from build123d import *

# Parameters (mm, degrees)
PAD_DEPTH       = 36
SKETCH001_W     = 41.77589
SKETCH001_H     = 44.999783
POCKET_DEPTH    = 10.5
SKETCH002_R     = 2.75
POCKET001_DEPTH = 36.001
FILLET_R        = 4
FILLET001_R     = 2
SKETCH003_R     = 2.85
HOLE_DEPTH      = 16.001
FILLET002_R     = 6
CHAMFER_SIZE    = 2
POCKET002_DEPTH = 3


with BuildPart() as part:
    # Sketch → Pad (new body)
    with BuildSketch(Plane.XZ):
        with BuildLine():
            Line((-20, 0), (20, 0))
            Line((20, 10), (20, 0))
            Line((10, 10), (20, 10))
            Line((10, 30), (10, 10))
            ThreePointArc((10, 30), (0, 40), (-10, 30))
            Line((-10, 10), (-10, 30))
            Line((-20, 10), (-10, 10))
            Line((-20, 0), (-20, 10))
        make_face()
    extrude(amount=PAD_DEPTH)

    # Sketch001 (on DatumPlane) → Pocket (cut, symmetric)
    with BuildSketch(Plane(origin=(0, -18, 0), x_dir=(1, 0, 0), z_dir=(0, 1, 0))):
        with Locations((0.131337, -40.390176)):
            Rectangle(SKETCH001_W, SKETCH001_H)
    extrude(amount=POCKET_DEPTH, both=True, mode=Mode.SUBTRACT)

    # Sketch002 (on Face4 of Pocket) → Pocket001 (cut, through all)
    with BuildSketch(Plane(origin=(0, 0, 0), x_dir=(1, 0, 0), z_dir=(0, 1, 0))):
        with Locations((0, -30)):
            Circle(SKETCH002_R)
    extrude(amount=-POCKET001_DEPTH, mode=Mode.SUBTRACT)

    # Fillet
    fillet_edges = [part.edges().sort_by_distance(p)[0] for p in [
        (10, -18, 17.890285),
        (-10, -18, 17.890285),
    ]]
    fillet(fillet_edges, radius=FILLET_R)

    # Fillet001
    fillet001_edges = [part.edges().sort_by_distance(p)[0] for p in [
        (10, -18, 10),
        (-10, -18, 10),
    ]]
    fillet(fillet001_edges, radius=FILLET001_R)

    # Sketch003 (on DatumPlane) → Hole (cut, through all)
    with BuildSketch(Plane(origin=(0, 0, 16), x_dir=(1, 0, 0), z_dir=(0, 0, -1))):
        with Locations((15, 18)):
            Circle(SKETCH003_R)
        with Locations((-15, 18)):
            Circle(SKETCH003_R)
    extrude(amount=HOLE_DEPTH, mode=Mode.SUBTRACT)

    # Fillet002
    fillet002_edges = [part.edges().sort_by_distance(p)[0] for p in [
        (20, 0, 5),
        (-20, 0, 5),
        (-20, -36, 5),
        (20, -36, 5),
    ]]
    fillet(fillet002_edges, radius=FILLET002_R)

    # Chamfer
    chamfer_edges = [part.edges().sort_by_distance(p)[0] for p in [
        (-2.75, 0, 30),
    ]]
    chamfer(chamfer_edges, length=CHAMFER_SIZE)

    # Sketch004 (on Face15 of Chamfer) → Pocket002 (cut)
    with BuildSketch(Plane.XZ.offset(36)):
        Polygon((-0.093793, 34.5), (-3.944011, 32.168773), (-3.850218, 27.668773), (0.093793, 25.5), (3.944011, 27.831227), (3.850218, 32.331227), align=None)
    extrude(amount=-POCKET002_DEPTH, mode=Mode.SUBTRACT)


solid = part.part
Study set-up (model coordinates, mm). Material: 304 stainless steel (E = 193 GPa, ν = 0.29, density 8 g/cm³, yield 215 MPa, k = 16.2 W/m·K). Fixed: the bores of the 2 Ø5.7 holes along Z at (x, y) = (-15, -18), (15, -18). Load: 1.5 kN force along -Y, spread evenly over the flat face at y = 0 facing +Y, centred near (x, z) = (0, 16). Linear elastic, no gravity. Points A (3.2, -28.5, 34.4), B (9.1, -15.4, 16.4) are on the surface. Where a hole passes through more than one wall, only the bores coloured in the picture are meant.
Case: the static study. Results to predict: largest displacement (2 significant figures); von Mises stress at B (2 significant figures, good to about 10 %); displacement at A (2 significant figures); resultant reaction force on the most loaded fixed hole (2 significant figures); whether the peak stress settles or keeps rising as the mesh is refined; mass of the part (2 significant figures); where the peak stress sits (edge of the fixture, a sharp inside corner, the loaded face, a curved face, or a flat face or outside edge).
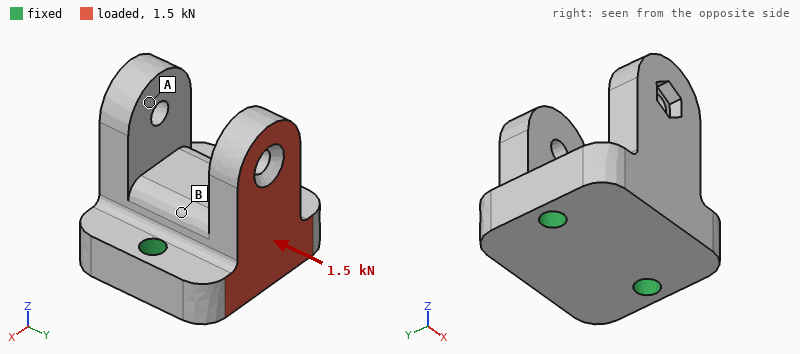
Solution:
19 µm
8.6 MPa
3.8 µm
750 N
keeps rising
200 g
edge of the fixture
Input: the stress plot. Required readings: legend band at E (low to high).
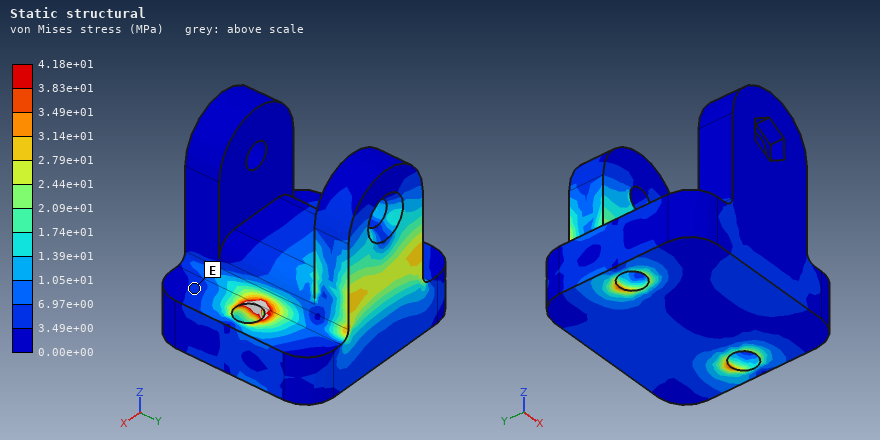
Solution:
3.49e+00 to 6.97e+00 MPa
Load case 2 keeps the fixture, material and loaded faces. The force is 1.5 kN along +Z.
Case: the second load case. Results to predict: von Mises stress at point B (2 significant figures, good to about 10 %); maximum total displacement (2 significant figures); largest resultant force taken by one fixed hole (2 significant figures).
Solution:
9.3 MPa
16 µm
800 N
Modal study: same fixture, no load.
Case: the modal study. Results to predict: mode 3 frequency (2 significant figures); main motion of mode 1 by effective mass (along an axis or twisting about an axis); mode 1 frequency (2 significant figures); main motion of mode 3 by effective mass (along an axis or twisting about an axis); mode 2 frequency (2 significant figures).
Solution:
12 kHz
along Y
6700 Hz
along X
9100 Hz
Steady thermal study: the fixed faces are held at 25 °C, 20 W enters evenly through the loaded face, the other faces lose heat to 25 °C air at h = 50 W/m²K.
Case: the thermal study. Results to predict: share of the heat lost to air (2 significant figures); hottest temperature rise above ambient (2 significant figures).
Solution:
29 %
74 K
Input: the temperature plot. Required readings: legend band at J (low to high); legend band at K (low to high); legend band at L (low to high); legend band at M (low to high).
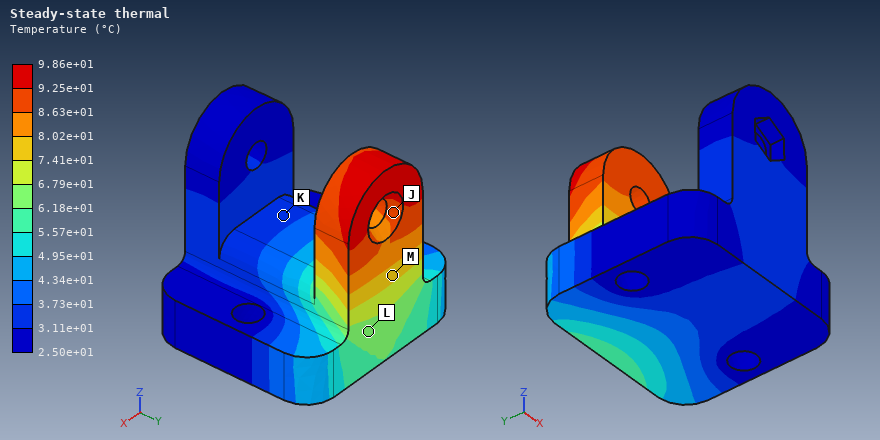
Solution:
8.63e+01 to 9.25e+01 °C
3.11e+01 to 3.73e+01 °C
6.18e+01 to 6.79e+01 °C
7.41e+01 to 8.02e+01 °C
